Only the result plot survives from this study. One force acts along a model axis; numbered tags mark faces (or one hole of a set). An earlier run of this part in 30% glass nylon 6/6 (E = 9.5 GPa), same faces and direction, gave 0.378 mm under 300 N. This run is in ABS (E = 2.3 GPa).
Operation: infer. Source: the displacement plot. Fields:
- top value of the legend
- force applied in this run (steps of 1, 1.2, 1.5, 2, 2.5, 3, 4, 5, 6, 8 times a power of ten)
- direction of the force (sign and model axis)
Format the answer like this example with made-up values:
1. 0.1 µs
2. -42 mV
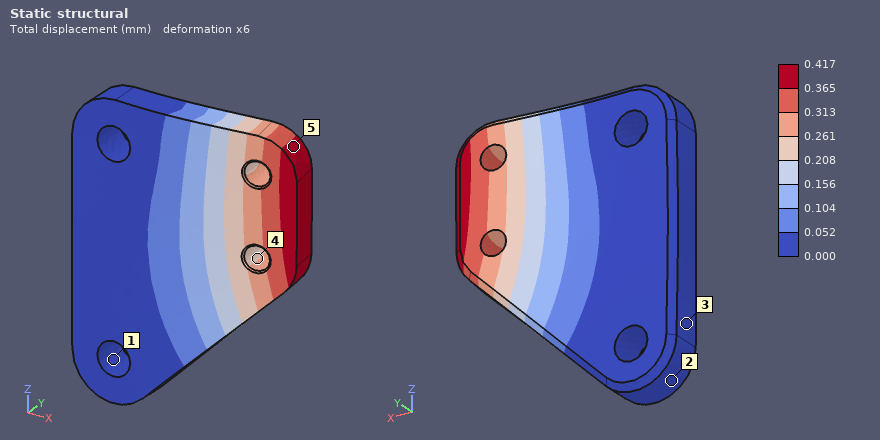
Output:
1. 0.417 mm
2. 80 N
3. +Y
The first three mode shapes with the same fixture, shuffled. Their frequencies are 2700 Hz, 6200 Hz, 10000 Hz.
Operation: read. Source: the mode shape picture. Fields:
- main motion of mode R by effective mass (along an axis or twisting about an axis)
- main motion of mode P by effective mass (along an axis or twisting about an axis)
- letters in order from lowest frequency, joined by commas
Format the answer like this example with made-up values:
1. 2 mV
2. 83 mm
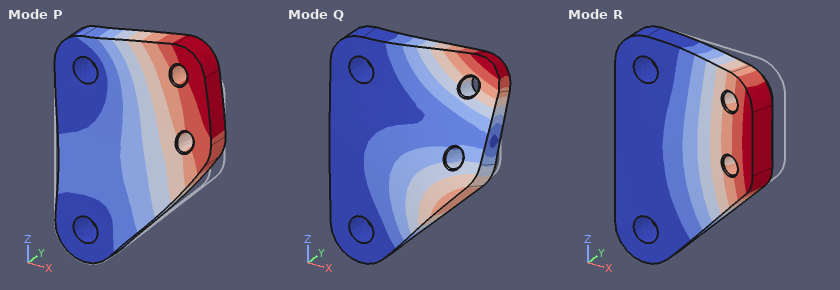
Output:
1. along Y
2. along Z
3. R, Q, P
